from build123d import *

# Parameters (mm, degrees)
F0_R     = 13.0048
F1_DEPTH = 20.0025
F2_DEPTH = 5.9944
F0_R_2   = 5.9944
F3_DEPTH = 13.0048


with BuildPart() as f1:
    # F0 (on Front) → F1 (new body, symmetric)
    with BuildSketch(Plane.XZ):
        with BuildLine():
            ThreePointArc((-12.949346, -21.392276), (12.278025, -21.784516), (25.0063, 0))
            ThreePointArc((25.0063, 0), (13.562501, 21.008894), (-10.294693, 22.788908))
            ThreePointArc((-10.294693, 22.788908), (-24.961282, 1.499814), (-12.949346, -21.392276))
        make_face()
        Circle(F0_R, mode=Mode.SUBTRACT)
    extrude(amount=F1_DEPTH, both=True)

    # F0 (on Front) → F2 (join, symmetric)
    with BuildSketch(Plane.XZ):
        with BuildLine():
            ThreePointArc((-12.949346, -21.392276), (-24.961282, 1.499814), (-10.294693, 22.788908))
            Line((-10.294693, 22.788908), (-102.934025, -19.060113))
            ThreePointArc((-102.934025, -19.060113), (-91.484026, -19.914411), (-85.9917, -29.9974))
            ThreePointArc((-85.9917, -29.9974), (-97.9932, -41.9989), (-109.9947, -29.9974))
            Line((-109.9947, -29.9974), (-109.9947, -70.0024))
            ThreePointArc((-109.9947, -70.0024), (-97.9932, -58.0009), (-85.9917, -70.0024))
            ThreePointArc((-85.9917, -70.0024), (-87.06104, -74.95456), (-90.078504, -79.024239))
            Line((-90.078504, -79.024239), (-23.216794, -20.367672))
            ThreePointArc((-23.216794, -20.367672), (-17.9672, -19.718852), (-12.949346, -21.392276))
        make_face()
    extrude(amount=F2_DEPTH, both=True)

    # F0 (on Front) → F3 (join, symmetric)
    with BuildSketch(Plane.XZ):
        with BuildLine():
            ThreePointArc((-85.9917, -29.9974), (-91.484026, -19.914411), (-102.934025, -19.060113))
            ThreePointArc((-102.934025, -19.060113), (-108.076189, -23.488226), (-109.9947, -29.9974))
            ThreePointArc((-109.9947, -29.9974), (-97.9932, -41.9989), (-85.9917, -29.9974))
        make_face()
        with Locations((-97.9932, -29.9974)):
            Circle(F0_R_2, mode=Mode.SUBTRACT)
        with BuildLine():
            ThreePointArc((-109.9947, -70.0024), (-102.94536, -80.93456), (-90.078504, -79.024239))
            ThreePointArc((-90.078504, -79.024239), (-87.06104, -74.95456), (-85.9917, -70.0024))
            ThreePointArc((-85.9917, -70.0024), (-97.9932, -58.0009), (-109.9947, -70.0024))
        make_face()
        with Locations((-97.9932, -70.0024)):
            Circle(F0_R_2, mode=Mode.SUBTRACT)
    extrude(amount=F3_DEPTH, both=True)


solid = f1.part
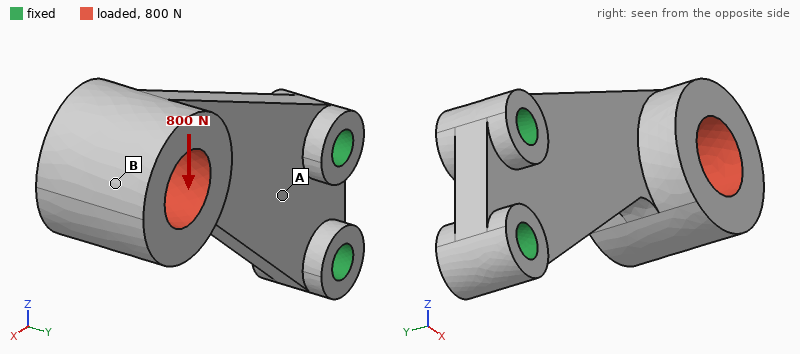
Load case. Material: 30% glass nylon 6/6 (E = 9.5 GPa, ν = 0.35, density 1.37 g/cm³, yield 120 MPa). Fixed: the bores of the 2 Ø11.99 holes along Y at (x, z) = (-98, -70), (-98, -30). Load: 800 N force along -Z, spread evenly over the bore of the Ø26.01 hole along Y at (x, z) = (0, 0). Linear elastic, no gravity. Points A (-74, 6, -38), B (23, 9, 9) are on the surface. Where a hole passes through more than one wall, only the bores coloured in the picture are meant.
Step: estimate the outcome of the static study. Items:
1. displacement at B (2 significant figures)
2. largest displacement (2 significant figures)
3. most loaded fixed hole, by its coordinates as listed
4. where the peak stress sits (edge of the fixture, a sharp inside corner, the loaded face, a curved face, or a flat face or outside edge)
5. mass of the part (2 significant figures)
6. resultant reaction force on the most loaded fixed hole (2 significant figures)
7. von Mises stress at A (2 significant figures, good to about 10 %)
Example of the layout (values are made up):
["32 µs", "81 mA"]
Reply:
["0.47 mm", "0.47 mm", "(-98, -70)", "a curved face", "170 g", "1.9 kN", "4.1 MPa"]
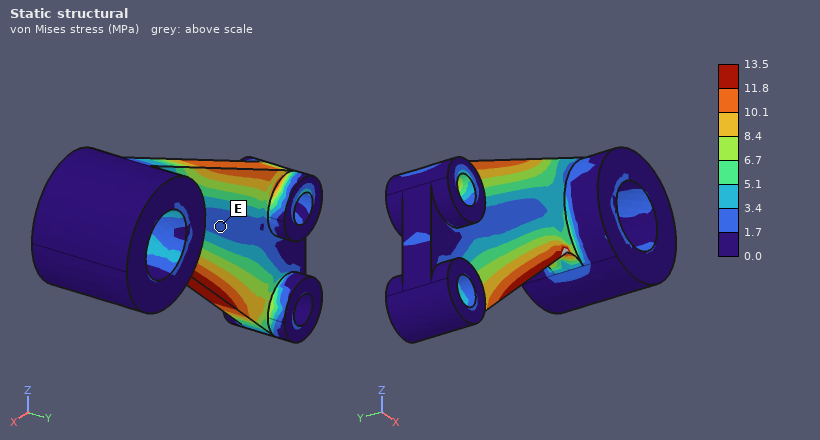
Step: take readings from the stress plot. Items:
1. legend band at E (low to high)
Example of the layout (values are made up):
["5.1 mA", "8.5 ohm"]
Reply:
["1.7 to 3.4 MPa"]
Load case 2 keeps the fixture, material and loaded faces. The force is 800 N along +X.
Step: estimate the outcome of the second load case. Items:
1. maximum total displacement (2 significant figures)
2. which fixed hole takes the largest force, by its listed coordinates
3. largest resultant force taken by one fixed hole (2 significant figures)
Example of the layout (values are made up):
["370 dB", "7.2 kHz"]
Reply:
["0.17 mm", "(-98, -30)", "1.3 kN"]
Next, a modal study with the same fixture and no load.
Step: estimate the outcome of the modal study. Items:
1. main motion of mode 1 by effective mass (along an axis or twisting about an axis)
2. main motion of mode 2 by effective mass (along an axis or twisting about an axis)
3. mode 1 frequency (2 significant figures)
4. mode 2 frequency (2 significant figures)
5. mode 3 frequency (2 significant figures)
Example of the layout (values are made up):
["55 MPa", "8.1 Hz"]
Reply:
["along Y", "along Z", "240 Hz", "780 Hz", "950 Hz"]
